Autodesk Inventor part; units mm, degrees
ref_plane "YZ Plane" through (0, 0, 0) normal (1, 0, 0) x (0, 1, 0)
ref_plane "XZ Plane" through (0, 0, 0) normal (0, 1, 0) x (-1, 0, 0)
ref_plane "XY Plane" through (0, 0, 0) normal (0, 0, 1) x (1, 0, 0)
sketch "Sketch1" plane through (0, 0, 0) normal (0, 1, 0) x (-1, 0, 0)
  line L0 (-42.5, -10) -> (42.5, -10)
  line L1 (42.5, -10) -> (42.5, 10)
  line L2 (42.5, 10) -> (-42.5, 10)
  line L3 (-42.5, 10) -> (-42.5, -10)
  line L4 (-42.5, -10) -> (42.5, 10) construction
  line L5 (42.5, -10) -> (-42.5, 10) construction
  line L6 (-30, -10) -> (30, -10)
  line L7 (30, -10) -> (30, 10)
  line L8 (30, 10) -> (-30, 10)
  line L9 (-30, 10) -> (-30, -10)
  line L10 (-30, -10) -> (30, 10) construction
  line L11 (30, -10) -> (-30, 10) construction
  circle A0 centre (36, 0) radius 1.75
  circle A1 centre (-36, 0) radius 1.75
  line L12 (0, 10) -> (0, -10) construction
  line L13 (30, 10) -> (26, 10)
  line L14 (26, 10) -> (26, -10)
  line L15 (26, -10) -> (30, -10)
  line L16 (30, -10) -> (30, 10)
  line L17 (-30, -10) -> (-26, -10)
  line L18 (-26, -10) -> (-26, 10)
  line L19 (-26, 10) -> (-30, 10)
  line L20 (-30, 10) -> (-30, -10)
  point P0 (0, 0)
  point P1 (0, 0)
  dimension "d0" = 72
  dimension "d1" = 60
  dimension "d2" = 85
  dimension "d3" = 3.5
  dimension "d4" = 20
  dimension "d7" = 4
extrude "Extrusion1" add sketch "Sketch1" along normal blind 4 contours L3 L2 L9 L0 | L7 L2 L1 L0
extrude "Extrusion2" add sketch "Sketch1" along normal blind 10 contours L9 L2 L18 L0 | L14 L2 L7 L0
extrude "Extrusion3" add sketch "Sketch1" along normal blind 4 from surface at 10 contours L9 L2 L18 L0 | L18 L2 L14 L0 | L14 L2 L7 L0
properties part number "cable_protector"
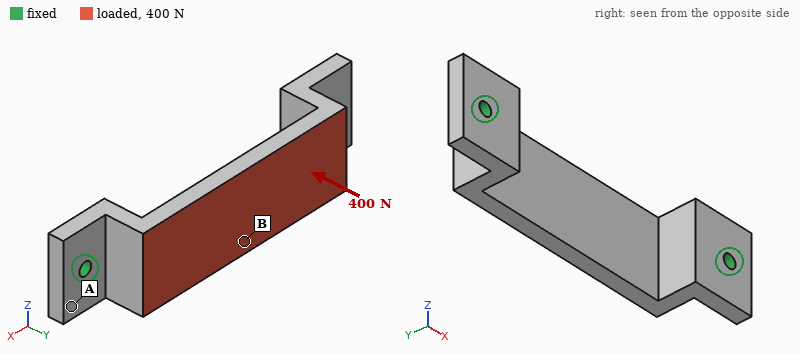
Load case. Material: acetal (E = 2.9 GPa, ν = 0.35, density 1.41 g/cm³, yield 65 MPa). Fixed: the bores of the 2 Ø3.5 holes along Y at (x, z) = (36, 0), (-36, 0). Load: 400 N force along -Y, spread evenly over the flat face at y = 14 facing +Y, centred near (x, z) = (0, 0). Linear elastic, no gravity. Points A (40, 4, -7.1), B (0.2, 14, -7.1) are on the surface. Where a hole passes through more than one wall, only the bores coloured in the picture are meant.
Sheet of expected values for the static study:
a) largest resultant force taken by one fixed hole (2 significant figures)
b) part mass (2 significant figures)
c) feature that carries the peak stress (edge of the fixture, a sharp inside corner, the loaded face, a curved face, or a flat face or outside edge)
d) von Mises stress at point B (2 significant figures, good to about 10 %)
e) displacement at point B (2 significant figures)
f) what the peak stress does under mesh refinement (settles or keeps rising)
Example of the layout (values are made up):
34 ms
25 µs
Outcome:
320 N
12 g
edge of the fixture
21 MPa
0.75 mm
keeps rising
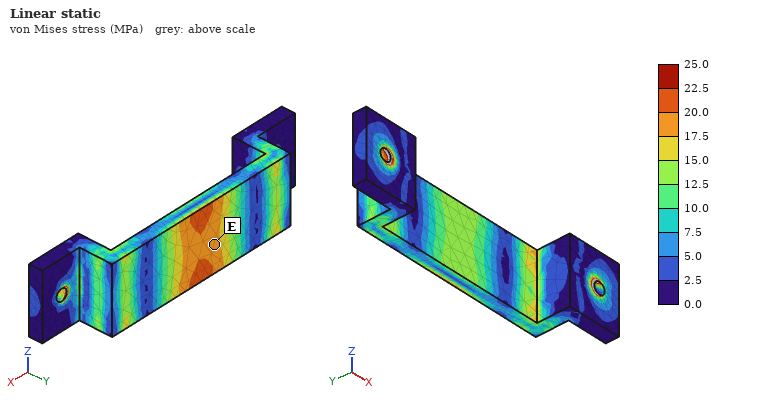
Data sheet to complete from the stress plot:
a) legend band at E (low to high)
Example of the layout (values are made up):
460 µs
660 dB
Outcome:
17.5 to 20.0 MPa
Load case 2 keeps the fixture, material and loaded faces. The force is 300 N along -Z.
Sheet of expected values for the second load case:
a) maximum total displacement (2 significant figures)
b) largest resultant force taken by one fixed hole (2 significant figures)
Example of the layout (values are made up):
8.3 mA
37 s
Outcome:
0.65 mm
150 N
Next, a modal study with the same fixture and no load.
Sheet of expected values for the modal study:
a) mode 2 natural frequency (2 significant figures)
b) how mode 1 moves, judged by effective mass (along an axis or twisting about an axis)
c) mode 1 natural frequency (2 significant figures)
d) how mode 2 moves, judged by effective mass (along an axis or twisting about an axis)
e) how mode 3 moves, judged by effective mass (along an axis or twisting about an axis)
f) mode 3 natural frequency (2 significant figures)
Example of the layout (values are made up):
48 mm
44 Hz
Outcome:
1600 Hz
along Z
1500 Hz
along Y
along X
1900 Hz
